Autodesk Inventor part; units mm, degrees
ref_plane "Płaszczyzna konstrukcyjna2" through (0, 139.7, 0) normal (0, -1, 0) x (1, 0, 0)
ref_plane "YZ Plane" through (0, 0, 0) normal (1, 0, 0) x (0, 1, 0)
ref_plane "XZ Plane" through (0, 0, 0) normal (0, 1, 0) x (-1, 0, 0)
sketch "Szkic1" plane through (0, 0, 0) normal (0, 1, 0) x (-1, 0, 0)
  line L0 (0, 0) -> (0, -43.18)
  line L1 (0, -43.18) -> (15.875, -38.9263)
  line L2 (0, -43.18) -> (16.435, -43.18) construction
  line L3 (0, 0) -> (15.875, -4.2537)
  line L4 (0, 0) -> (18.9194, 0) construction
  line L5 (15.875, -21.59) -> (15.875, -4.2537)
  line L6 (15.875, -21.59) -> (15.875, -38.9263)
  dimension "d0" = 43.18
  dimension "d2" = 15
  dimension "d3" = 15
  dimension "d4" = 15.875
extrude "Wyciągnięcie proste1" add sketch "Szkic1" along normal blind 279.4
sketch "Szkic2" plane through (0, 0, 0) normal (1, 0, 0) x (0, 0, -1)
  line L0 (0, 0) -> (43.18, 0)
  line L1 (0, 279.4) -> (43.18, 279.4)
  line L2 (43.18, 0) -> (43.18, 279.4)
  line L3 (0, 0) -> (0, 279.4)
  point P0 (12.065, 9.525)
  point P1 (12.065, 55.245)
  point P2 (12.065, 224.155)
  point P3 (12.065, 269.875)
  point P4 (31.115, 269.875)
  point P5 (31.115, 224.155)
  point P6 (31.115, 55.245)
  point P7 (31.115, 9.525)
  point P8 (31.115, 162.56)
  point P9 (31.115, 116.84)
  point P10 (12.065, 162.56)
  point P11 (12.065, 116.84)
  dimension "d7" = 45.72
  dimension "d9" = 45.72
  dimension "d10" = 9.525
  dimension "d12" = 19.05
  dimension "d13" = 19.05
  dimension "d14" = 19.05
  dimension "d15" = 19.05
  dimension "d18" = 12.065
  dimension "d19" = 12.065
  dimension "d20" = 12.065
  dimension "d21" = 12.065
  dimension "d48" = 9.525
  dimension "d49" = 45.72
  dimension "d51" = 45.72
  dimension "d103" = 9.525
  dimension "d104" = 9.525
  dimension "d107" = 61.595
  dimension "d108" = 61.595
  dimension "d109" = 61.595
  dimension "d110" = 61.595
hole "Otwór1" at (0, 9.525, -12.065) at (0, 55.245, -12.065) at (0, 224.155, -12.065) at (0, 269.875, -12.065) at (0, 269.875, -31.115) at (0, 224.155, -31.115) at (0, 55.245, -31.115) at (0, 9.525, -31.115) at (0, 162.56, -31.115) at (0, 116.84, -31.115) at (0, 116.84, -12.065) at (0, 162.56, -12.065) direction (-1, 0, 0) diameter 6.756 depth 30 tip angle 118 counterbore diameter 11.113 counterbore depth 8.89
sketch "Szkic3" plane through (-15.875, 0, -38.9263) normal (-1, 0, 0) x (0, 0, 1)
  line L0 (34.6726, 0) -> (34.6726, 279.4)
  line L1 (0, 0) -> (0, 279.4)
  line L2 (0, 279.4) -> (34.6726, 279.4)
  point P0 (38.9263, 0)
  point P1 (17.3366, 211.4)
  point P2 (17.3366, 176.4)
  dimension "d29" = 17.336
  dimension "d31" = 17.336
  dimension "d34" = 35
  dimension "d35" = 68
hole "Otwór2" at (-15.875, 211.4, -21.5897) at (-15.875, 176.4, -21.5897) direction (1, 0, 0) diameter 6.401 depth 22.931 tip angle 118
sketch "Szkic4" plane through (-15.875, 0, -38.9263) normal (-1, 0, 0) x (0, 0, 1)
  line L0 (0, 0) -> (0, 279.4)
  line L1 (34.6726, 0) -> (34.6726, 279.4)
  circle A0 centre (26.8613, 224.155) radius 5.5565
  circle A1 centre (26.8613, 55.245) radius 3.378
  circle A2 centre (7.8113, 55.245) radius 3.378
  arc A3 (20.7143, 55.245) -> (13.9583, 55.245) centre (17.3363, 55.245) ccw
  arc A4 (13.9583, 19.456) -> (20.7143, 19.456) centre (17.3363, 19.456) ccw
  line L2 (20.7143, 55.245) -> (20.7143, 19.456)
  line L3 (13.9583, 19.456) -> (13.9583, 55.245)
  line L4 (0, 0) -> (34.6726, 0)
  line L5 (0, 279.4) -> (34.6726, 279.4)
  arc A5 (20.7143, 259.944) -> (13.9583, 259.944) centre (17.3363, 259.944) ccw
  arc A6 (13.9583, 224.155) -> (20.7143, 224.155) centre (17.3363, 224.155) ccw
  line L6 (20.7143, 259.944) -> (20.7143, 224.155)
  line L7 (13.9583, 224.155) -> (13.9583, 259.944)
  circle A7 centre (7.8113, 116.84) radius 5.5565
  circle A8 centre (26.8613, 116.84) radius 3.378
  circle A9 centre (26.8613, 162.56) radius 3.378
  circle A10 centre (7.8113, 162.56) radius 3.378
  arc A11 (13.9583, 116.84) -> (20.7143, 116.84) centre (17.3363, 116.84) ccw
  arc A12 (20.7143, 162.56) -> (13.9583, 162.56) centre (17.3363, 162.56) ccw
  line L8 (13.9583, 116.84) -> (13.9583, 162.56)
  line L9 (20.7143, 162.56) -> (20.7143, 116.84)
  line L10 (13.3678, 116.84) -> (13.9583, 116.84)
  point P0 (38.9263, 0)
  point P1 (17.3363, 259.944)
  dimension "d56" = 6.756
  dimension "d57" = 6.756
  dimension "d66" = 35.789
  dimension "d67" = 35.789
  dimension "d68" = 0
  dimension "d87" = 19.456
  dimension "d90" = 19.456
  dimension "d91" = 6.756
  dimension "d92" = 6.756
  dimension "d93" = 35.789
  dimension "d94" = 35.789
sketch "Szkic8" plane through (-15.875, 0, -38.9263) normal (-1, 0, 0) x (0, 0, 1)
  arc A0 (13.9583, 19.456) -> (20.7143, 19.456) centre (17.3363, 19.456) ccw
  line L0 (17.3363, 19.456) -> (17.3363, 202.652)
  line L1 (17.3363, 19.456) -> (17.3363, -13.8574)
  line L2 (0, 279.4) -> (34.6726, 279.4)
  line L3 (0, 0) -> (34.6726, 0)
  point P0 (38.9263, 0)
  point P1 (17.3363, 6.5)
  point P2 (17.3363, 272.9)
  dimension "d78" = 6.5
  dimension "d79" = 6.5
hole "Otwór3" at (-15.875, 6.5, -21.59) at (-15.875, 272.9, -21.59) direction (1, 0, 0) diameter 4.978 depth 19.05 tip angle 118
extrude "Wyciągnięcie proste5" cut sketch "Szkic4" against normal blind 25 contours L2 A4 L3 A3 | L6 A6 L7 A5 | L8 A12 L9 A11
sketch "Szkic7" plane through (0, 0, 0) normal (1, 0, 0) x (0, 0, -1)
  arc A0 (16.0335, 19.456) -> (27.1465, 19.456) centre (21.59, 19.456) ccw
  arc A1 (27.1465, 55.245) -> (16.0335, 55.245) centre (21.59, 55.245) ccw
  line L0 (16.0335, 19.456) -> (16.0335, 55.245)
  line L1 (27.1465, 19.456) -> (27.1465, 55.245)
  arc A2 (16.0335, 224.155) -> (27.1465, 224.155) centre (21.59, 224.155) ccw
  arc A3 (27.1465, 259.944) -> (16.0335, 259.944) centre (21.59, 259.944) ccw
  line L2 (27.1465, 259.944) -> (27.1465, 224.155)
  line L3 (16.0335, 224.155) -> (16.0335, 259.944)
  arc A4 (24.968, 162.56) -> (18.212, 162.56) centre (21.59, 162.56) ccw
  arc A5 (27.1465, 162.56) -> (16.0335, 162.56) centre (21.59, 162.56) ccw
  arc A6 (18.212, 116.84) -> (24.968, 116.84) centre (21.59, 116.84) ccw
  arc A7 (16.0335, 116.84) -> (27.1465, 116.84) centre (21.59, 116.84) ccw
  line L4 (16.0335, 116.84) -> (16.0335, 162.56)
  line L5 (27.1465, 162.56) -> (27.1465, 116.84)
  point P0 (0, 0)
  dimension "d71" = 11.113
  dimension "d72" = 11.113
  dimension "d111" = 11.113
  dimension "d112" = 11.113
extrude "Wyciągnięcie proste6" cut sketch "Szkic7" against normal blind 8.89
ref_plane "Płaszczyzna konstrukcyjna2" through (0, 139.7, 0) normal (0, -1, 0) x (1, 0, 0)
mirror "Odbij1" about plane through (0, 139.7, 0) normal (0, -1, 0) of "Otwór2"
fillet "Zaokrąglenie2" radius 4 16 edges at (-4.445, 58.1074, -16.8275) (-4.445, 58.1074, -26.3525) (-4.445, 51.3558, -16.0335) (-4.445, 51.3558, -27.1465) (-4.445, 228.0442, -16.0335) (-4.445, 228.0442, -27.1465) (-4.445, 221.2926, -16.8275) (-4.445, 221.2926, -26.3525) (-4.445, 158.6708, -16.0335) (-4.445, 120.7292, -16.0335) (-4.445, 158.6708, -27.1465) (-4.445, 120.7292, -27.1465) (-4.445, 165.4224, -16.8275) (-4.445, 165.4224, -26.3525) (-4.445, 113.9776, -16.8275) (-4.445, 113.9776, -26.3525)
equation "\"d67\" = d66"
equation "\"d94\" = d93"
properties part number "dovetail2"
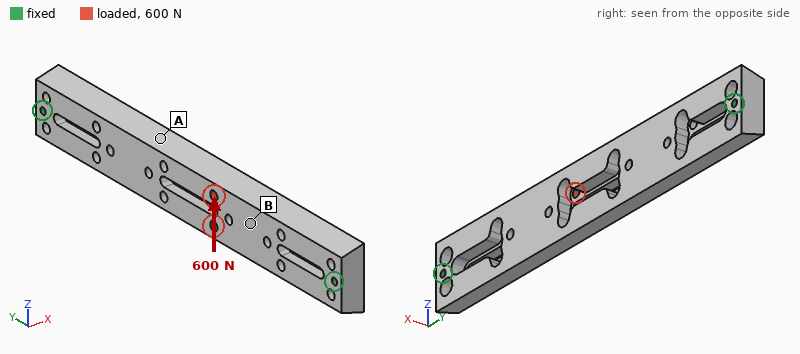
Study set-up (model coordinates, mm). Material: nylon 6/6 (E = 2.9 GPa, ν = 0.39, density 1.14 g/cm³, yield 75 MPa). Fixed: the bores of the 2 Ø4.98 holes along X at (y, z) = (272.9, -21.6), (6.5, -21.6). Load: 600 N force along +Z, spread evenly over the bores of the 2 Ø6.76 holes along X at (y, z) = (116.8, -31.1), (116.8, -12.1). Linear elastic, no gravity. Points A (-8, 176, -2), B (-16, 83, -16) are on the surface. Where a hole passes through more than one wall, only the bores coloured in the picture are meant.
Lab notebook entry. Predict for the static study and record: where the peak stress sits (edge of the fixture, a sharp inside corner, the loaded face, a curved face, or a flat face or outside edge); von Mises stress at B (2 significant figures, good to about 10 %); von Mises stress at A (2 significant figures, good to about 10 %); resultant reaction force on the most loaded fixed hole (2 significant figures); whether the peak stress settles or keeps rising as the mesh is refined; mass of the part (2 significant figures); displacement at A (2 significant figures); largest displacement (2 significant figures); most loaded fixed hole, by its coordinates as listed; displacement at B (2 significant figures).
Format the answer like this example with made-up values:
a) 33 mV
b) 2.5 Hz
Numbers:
a) edge of the fixture
b) 2.4 MPa
c) 4.0 MPa
d) 360 N
e) keeps rising
f) 160 g
g) 0.84 mm
h) 1.2 mm
i) (6.5, -21.6)
j) 0.98 mm
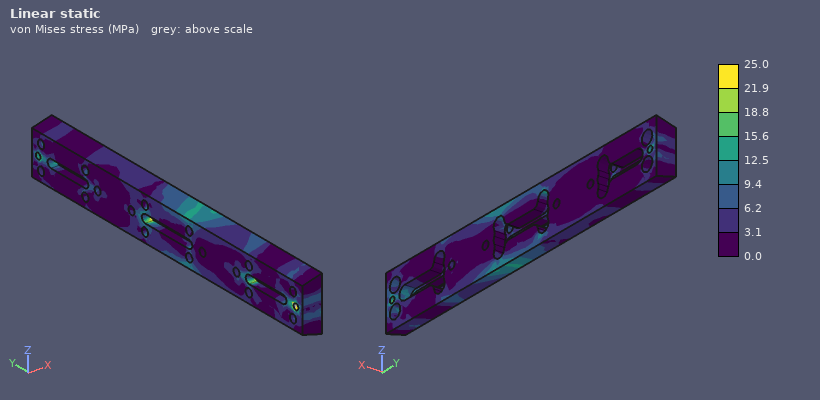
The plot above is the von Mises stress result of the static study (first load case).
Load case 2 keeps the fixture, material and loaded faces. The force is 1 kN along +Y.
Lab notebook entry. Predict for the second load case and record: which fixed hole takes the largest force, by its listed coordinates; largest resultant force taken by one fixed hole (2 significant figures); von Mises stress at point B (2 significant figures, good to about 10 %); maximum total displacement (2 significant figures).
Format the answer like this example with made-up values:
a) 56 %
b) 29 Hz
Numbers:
a) (6.5, -21.6)
b) 580 N
c) 1.9 MPa
d) 0.15 mm
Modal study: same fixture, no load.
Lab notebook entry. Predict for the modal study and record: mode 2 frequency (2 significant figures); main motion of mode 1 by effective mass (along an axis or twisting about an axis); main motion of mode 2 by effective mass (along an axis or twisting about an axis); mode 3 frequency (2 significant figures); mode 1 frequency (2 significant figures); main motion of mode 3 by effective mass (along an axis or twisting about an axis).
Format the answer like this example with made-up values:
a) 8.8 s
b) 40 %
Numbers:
a) 420 Hz
b) along X
c) along Z
d) 750 Hz
e) 280 Hz
f) twisting about Z
